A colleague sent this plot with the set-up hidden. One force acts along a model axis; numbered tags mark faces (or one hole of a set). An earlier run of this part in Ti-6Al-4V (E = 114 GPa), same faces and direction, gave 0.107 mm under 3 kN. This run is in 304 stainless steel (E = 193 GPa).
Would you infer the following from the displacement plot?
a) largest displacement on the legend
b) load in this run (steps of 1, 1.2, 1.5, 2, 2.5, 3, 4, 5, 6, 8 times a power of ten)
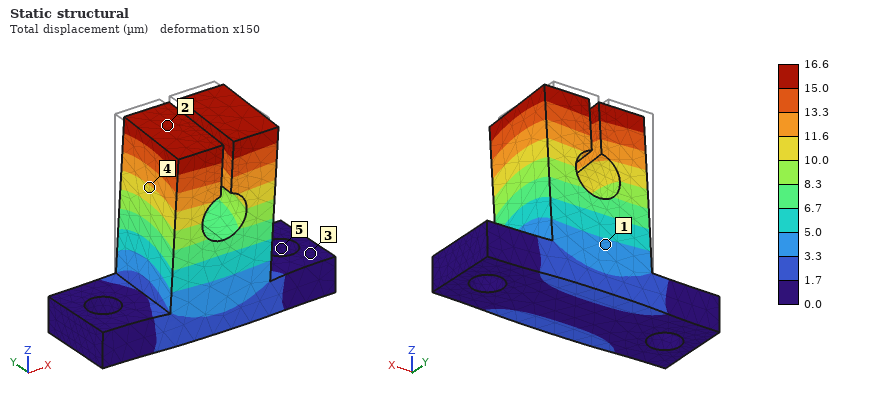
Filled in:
16.6 µm
800 N
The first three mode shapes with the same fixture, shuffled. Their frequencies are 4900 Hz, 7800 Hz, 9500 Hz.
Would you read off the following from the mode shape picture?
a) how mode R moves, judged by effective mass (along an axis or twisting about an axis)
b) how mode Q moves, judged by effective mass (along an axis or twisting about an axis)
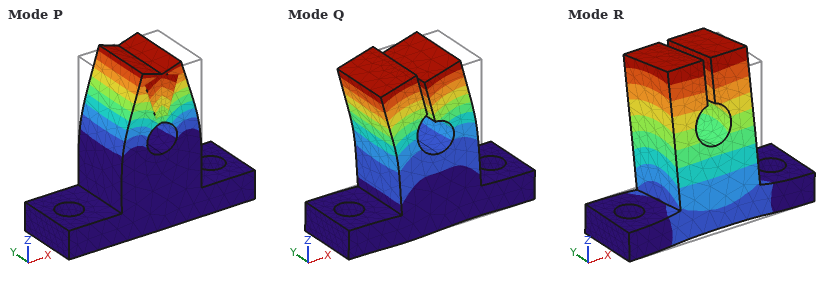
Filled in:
along Y
along X
